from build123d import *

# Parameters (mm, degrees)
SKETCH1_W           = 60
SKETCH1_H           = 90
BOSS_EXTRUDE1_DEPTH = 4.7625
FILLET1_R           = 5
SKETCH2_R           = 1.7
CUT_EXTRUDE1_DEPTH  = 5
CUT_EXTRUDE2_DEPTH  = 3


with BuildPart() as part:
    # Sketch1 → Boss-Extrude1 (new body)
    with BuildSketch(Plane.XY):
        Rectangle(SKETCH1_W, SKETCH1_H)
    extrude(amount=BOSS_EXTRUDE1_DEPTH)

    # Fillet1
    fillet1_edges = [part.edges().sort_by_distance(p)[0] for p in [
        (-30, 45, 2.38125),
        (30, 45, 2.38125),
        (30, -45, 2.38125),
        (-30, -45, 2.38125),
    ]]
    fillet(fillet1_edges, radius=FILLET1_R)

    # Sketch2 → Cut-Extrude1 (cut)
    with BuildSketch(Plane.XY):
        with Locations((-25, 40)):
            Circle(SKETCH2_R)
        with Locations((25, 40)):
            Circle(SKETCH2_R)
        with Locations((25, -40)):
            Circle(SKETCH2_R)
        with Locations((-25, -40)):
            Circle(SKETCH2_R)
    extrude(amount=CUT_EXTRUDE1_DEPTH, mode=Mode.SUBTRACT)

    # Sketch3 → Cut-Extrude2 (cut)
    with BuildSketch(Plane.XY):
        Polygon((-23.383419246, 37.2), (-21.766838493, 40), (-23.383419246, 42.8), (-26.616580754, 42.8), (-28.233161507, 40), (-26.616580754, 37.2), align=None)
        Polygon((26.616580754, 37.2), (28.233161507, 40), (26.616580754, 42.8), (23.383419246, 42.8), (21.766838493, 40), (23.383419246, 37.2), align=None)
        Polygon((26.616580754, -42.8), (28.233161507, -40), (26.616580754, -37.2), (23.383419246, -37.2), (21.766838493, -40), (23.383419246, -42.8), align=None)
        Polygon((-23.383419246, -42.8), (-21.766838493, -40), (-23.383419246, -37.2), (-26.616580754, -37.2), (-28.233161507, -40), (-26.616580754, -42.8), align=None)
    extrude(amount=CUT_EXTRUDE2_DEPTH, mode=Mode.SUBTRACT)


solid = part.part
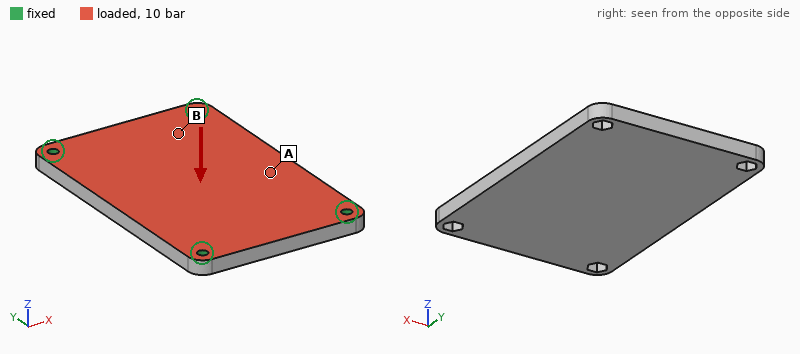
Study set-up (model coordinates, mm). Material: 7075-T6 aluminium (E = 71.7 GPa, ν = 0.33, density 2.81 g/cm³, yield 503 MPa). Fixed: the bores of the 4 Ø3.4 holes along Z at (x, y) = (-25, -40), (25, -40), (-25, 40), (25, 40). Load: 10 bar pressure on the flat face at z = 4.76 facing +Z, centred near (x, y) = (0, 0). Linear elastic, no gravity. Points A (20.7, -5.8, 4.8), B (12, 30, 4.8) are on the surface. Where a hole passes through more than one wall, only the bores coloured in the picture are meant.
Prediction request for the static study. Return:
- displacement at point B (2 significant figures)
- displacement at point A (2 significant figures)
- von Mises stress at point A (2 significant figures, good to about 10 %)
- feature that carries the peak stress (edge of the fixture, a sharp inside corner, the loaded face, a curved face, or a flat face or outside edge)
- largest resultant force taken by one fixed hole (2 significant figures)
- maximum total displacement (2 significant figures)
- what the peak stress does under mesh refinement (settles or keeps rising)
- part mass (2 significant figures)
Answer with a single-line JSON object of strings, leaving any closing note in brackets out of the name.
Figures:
{"displacement at point B": "0.16 mm", "displacement at point A": "0.37 mm", "von Mises stress at point A": "91 MPa", "feature that carries the peak stress": "edge of the fixture", "largest resultant force taken by one fixed hole": "2.8 kN", "maximum total displacement": "0.39 mm", "what the peak stress does under mesh refinement": "keeps rising", "part mass": "71 g"}
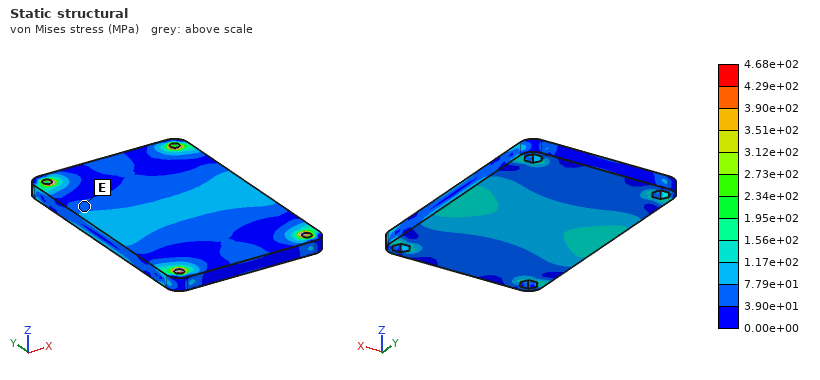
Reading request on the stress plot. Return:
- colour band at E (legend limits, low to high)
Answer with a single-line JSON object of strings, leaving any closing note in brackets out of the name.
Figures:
{"colour band at E": "3.90e+01 to 7.79e+01 MPa"}
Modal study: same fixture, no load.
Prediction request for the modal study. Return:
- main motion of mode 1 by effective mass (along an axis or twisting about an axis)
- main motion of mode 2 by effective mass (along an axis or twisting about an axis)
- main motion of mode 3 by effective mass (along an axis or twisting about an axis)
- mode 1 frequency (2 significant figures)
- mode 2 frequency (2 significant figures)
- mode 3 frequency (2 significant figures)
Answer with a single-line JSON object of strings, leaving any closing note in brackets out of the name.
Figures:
{"main motion of mode 1 by effective mass": "along Z", "main motion of mode 2 by effective mass": "twisting about Y", "main motion of mode 3 by effective mass": "twisting about X", "mode 1 frequency": "2500 Hz", "mode 2 frequency": "4200 Hz", "mode 3 frequency": "6400 Hz"}
